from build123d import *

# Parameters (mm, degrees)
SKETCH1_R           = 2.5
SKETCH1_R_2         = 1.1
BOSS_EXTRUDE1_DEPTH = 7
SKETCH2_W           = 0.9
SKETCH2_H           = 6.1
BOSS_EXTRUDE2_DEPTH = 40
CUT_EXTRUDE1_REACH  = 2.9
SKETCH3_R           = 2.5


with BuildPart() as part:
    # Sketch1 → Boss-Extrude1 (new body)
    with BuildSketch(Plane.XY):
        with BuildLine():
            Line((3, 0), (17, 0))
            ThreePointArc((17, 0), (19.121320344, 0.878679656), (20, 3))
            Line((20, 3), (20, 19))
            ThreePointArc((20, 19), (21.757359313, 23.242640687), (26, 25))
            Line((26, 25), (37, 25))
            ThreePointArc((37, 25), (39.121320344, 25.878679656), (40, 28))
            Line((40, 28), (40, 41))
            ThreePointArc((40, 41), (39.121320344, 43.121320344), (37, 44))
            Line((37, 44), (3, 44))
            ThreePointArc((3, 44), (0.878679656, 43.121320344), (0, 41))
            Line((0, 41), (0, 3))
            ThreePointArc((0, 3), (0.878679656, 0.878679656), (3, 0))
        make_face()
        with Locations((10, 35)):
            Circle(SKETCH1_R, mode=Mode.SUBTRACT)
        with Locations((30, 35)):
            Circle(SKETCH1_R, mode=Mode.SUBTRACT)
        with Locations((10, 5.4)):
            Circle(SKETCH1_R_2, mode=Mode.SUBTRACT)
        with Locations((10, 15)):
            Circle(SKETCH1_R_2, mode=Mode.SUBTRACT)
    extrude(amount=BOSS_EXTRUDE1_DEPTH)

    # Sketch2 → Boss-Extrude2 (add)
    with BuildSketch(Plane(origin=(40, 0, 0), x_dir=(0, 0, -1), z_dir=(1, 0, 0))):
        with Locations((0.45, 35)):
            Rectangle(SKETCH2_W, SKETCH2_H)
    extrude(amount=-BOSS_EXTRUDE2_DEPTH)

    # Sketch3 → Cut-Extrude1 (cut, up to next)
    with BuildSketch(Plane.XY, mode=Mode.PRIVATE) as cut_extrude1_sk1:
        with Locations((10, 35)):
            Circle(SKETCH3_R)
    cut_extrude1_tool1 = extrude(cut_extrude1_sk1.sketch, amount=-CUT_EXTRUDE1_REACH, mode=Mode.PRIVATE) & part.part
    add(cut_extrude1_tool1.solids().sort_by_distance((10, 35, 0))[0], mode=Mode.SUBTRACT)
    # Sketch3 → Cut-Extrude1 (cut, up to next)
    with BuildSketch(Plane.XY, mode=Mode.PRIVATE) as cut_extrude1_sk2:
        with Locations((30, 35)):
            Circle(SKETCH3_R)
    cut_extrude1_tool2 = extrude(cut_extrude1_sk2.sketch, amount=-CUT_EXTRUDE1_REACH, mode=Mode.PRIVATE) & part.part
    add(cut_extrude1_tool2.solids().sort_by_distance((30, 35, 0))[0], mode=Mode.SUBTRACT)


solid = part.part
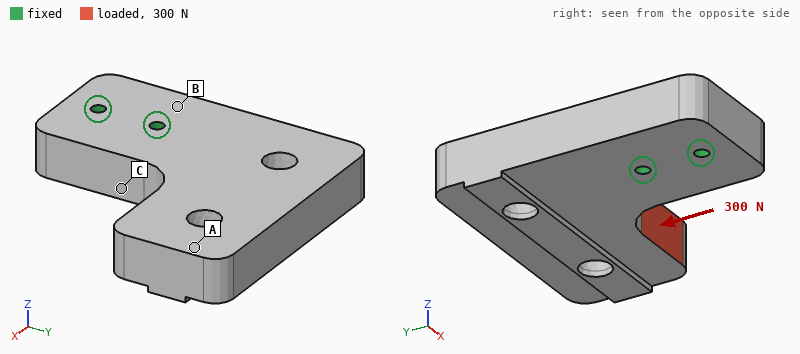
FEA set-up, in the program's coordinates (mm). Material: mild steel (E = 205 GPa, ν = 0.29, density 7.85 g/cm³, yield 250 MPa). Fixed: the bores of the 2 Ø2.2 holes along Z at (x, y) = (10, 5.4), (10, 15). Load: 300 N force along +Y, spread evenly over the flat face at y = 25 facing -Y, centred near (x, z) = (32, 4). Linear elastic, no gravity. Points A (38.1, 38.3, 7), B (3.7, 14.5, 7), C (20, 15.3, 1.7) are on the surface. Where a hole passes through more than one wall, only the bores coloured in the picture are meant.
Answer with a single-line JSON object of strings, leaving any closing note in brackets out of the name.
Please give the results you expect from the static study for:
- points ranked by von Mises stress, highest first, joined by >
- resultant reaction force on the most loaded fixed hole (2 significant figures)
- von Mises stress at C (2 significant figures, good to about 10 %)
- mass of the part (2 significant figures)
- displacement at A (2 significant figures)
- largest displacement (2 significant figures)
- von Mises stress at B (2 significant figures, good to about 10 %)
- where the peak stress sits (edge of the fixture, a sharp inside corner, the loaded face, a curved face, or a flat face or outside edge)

{"points ranked by von Mises stress, highest first, joined by >": "C > B > A", "resultant reaction force on the most loaded fixed hole": "590 N", "von Mises stress at C": "15 MPa", "mass of the part": "68 g", "displacement at A": "7.9 µm", "largest displacement": "8.7 µm", "von Mises stress at B": "7.9 MPa", "where the peak stress sits": "edge of the fixture"}
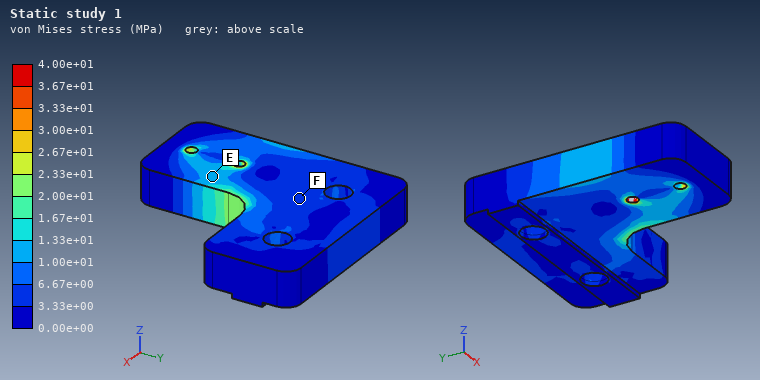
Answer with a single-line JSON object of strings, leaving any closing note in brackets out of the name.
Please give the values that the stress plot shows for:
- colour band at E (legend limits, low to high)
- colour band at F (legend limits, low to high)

{"colour band at E": "1.00e+01 to 1.33e+01 MPa", "colour band at F": "3.33e+00 to 6.67e+00 MPa"}
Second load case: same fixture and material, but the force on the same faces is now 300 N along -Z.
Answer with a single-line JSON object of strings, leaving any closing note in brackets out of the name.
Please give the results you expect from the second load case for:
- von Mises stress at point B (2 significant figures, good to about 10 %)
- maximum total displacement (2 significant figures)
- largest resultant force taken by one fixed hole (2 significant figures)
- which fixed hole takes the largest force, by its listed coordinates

{"von Mises stress at point B": "16 MPa", "maximum total displacement": "31 µm", "largest resultant force taken by one fixed hole": "390 N", "which fixed hole takes the largest force, by its listed coordinates": "(10, 15)"}
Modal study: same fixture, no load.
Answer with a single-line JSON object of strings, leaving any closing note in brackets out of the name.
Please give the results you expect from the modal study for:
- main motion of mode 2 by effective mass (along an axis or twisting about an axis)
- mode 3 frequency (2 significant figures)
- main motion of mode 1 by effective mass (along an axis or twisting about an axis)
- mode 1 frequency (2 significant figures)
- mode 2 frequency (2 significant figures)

{"main motion of mode 2 by effective mass": "along X", "mode 3 frequency": "6600 Hz", "main motion of mode 1 by effective mass": "along Z", "mode 1 frequency": "3400 Hz", "mode 2 frequency": "5800 Hz"}
